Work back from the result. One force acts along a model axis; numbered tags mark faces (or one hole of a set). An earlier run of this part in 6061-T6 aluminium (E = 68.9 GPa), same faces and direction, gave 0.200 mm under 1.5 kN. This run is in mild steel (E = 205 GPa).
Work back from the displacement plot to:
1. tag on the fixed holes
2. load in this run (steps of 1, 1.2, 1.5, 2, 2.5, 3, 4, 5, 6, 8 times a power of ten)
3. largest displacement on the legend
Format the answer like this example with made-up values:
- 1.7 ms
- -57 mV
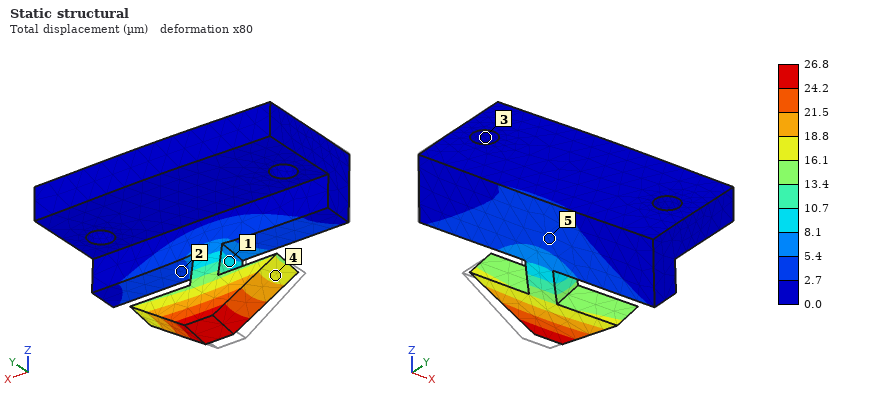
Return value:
- 3
- 600 N
- 26.8 µm
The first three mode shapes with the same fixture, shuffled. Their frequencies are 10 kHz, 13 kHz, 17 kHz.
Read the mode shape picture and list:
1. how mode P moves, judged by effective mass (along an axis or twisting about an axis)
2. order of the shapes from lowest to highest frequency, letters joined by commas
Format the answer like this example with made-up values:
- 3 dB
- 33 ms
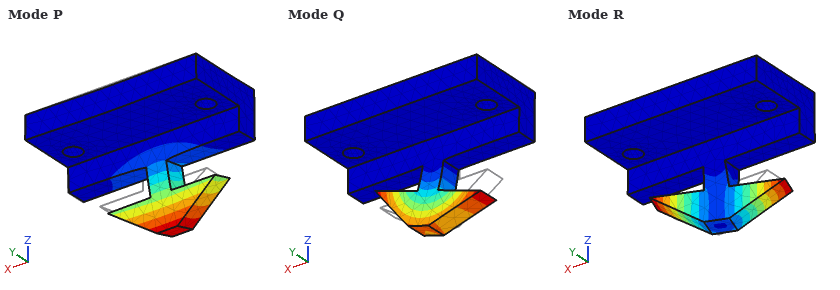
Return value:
- along Y
- P, Q, R
